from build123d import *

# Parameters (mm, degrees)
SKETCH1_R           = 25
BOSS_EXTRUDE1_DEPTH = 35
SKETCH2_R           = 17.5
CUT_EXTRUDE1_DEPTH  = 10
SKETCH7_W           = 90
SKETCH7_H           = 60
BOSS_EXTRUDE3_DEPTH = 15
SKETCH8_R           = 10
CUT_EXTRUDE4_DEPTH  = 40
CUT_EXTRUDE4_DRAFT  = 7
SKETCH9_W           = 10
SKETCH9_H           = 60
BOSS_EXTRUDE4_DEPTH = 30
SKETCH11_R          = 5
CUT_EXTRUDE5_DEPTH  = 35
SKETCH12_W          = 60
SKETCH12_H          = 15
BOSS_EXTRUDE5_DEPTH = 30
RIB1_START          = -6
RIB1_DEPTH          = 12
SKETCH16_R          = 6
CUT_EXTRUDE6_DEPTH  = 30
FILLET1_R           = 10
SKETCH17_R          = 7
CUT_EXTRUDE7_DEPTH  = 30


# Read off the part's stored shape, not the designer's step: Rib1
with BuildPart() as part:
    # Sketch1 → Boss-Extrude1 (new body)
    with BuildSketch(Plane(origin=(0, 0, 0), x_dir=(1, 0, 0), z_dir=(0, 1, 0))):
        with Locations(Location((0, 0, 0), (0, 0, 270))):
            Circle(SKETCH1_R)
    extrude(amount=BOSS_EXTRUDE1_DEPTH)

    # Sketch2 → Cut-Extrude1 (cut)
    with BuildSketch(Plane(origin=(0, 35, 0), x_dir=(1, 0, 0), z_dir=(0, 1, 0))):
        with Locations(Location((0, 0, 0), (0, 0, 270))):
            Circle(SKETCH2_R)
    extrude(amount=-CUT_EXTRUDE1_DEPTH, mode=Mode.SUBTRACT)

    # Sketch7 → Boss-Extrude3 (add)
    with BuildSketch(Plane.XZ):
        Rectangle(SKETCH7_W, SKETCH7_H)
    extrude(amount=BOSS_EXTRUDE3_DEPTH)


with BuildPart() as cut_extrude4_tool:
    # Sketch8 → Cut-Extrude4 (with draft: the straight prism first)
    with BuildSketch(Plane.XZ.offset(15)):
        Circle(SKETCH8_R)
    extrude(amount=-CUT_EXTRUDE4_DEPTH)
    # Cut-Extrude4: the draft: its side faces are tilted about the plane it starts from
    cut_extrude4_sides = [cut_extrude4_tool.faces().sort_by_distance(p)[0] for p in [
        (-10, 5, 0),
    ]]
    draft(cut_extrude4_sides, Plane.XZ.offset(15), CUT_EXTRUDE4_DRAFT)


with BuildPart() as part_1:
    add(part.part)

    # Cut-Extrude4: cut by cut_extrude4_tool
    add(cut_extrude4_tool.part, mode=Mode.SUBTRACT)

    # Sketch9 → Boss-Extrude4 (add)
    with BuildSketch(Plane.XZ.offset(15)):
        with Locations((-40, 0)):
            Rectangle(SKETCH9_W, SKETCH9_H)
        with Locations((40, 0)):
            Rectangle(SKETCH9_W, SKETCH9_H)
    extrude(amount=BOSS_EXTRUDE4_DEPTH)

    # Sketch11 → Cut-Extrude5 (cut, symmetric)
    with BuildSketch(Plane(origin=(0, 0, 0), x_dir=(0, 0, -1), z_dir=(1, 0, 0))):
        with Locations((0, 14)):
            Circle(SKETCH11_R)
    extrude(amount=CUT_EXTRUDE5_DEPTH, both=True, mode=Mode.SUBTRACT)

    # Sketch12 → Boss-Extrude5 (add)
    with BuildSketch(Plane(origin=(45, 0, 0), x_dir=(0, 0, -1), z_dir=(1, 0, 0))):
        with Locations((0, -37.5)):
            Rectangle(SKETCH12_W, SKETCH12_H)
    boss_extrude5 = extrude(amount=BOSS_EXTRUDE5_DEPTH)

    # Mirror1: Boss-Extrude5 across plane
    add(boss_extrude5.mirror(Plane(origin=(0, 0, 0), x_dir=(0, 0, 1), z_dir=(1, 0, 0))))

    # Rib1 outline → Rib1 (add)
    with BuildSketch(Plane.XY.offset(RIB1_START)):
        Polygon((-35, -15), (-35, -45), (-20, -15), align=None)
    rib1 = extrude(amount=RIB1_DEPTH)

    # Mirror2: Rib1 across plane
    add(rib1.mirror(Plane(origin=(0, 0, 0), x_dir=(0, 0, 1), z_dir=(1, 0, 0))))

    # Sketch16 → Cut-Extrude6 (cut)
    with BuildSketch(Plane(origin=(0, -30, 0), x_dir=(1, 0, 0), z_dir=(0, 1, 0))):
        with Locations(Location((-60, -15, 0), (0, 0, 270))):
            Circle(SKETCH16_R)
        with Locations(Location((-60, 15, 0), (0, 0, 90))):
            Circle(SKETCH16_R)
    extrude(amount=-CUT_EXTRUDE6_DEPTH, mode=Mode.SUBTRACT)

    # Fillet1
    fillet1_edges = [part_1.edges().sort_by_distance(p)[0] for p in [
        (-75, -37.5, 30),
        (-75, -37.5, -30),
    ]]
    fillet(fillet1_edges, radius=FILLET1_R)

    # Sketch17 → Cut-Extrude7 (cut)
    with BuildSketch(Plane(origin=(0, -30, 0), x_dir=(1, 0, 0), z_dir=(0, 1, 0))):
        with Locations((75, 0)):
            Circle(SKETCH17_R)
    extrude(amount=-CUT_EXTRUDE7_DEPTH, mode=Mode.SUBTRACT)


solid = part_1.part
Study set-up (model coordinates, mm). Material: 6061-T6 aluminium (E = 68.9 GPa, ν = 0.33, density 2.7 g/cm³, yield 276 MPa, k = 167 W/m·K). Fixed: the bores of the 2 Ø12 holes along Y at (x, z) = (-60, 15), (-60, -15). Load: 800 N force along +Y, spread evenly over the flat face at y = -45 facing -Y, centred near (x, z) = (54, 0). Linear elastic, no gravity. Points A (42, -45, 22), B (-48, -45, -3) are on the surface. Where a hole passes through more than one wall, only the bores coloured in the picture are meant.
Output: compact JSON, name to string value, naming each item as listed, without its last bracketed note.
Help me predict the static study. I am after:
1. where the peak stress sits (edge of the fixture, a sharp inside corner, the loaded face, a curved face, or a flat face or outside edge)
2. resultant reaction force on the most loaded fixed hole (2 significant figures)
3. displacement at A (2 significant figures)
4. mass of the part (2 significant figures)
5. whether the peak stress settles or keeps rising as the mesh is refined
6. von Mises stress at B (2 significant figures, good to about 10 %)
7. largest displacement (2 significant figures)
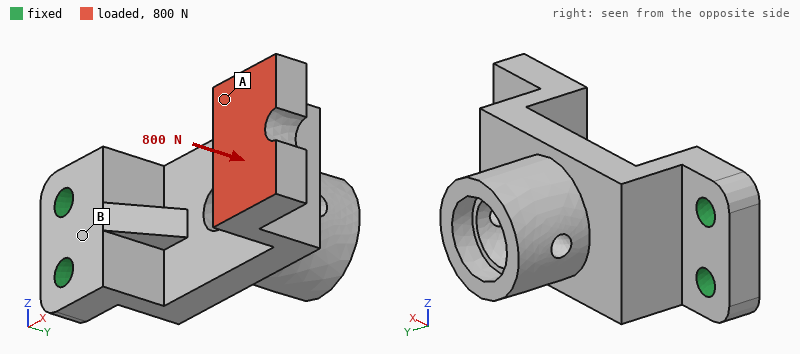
{"where the peak stress sits": "edge of the fixture", "resultant reaction force on the most loaded fixed hole": "430 N", "displacement at A": "0.38 mm", "mass of the part": "560 g", "whether the peak stress settles or keeps rising as the mesh is refined": "keeps rising", "von Mises stress at B": "33 MPa", "largest displacement": "0.54 mm"}
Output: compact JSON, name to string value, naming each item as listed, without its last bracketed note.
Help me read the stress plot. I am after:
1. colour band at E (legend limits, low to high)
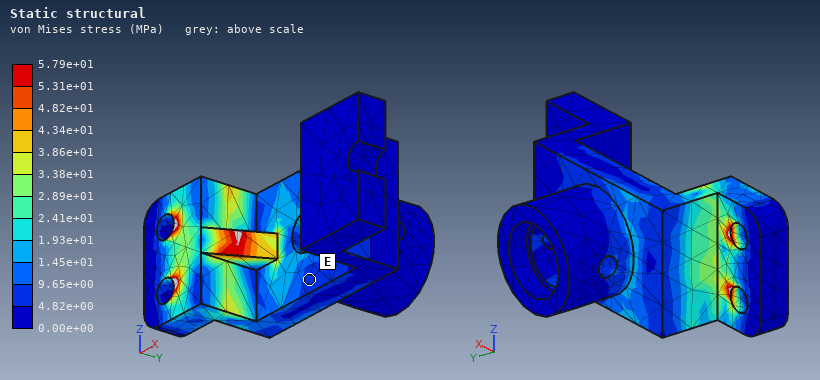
{"colour band at E": "4.82e+00 to 9.65e+00 MPa"}
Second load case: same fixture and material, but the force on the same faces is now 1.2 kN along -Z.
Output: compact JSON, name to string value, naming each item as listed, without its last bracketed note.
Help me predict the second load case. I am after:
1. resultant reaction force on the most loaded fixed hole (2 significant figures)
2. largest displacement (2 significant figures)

{"resultant reaction force on the most loaded fixed hole": "3.7 kN", "largest displacement": "0.33 mm"}
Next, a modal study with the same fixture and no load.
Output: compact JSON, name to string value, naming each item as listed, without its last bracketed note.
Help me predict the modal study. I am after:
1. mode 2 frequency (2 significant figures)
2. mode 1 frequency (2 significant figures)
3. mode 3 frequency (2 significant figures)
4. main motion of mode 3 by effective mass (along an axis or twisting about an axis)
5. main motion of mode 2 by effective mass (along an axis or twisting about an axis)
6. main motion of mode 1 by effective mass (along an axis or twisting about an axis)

{"mode 2 frequency": "860 Hz", "mode 1 frequency": "470 Hz", "mode 3 frequency": "2000 Hz", "main motion of mode 3 by effective mass": "along X", "main motion of mode 2 by effective mass": "along Z", "main motion of mode 1 by effective mass": "along Y"}
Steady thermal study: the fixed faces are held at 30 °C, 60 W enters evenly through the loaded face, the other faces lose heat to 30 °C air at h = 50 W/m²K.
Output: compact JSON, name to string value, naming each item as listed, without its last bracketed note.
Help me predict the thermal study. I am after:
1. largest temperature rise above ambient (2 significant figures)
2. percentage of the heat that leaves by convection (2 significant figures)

{"largest temperature rise above ambient": "40 K", "percentage of the heat that leaves by convection": "53 %"}
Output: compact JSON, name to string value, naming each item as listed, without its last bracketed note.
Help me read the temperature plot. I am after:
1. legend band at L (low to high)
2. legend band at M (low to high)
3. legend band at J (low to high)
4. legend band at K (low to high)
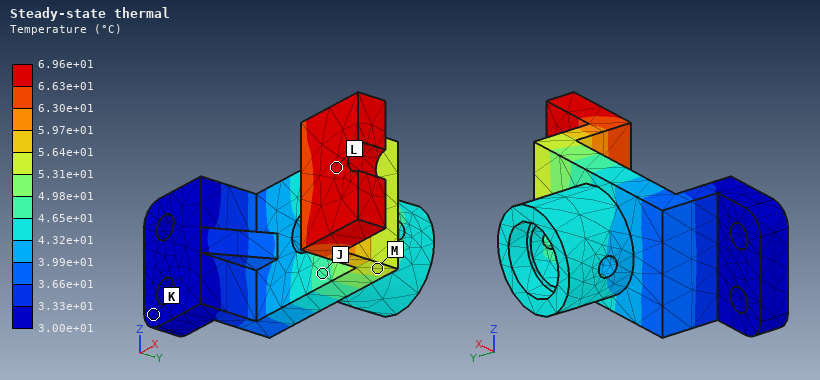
{"legend band at L": "6.63e+01 to 6.96e+01 °C", "legend band at M": "5.31e+01 to 5.64e+01 °C", "legend band at J": "4.65e+01 to 4.98e+01 °C", "legend band at K": "3.00e+01 to 3.33e+01 °C"}
